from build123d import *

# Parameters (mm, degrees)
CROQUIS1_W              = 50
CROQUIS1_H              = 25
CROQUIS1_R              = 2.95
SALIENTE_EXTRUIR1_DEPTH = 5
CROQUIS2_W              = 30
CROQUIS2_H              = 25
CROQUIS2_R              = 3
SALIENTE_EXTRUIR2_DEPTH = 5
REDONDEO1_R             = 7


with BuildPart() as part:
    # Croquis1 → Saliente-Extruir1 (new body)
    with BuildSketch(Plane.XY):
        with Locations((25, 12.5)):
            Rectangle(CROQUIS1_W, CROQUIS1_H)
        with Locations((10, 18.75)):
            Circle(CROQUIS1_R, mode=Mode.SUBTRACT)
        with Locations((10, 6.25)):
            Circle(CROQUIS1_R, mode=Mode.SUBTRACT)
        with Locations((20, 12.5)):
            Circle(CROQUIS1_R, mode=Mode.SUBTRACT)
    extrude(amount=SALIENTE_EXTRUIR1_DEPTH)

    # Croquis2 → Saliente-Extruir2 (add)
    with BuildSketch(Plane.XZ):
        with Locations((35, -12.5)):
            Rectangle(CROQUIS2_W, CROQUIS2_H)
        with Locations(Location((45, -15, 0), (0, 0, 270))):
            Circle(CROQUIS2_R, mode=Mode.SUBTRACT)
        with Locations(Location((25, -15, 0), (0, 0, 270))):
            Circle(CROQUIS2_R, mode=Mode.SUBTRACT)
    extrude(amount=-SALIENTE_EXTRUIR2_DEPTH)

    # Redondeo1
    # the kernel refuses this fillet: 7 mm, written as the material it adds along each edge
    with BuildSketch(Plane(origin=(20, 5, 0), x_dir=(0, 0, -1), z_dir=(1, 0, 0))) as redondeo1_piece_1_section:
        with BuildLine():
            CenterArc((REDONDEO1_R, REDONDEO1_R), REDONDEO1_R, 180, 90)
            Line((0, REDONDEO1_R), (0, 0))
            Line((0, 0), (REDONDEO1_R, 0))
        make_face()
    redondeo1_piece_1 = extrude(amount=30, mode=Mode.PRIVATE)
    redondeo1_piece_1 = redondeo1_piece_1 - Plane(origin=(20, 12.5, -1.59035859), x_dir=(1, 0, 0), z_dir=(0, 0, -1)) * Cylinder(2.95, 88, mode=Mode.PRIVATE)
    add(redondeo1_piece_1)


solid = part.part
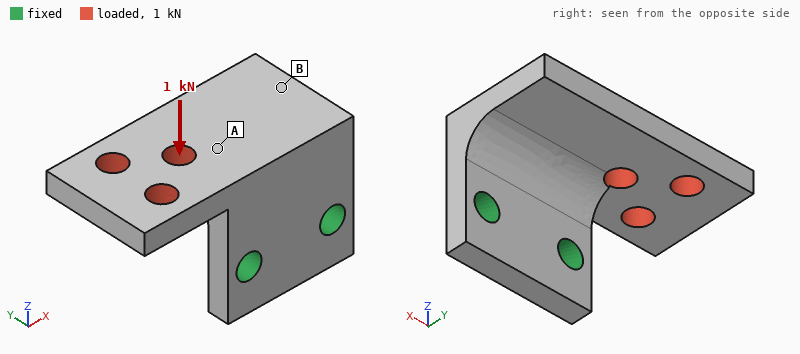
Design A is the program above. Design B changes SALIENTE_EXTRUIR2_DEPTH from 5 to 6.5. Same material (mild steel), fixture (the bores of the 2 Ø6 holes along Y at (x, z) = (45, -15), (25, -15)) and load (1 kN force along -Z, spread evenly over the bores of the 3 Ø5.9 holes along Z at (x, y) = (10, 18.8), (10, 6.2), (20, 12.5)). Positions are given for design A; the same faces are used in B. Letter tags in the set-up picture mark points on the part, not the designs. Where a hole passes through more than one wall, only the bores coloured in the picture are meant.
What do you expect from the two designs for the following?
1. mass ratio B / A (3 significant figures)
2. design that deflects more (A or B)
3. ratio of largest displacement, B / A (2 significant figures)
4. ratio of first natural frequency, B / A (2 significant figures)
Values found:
1.09
A
0.78
1.3
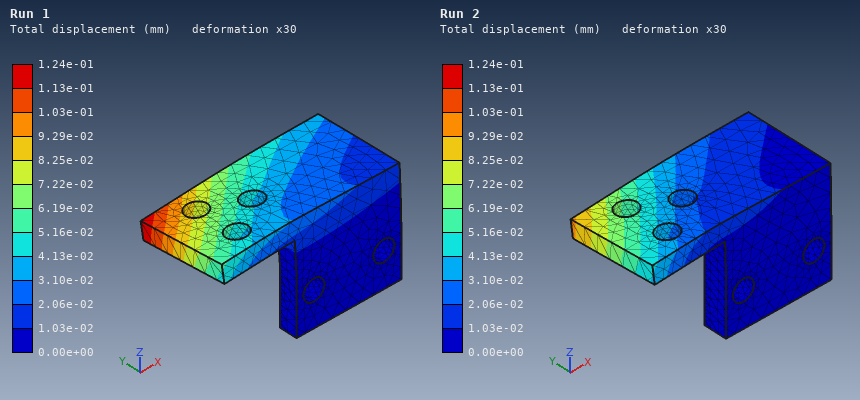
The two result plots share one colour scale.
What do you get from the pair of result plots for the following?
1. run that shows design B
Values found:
Run 2
